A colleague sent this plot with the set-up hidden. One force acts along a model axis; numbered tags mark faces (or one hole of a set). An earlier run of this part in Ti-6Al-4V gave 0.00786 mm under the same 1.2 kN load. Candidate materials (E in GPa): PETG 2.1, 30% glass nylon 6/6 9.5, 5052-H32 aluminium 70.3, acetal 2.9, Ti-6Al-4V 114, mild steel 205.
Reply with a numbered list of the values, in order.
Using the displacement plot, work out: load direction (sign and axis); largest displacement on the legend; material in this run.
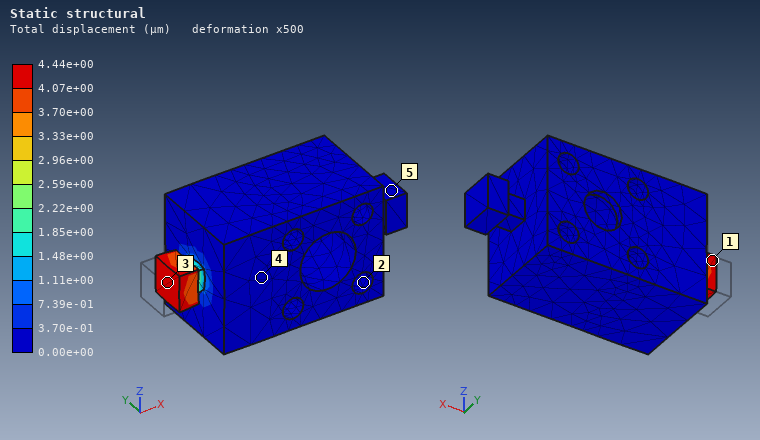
1. +X
2. 4.44e+00 µm
3. mild steel
